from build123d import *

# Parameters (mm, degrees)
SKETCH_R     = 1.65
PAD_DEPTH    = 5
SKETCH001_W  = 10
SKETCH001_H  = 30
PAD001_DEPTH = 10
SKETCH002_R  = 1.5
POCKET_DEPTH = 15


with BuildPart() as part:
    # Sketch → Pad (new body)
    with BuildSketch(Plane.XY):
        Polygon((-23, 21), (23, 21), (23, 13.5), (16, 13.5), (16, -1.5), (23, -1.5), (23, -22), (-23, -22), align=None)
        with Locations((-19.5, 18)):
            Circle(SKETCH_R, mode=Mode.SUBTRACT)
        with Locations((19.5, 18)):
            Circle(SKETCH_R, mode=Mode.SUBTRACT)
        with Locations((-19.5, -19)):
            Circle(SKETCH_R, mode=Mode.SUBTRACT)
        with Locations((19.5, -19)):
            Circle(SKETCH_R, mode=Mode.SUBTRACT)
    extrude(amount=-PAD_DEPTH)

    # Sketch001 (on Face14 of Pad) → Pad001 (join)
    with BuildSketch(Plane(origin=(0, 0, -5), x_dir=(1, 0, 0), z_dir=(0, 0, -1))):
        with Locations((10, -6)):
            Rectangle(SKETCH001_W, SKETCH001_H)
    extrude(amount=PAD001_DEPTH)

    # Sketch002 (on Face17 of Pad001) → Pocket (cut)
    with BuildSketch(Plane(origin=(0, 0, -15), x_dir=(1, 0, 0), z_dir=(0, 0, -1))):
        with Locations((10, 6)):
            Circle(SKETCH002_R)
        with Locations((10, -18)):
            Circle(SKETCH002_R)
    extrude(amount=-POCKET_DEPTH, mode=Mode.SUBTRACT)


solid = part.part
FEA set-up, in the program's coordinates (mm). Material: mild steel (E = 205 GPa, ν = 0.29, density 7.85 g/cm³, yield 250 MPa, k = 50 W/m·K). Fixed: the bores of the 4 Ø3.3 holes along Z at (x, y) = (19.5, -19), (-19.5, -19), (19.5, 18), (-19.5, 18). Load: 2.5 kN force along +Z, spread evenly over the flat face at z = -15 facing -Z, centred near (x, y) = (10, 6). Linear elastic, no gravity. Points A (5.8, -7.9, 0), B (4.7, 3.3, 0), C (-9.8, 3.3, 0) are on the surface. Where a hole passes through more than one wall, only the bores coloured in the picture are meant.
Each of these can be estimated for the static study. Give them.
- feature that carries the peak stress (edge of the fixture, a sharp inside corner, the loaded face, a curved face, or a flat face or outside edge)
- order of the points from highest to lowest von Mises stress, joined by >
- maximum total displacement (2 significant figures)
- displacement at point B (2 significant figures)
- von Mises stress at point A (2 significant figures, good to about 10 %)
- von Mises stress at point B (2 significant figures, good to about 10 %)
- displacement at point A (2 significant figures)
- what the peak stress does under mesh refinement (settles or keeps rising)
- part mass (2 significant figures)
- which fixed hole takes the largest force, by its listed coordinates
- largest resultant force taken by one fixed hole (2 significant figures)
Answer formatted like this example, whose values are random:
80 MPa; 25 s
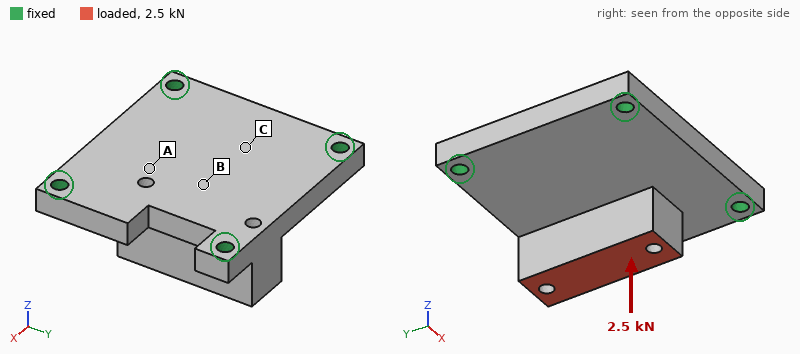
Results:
edge of the fixture; A > B > C; 12 µm; 10 µm; 43 MPa; 33 MPa; 9.8 µm; keeps rising; 94 g; (19.5, 18); 1.4 kN
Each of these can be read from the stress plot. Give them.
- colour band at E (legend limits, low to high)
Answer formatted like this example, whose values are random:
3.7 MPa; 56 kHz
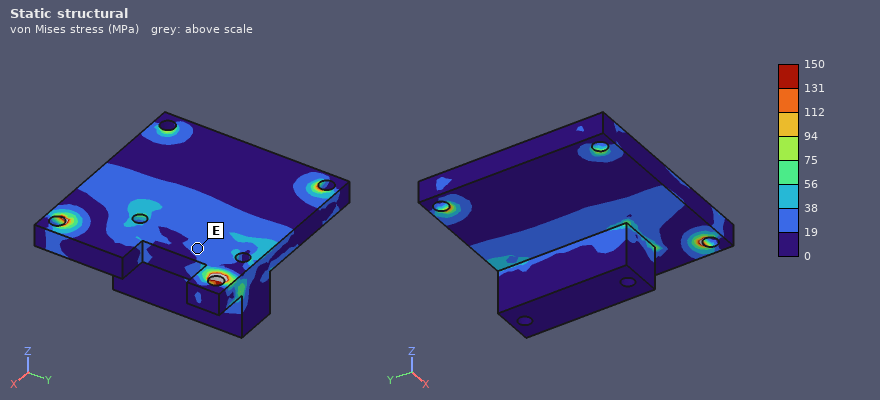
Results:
19 to 38 MPa
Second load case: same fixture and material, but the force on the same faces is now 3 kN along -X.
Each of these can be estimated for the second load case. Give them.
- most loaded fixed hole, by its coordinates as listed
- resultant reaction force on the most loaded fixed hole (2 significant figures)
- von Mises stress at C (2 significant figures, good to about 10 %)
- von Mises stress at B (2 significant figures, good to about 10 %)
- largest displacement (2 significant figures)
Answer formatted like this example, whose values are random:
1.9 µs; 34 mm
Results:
(19.5, 18); 1.4 kN; 23 MPa; 89 MPa; 30 µm
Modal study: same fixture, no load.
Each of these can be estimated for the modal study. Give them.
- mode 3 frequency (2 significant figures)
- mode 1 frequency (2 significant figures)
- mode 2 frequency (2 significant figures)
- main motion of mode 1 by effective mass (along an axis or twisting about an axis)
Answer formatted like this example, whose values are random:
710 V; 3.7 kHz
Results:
19 kHz; 9600 Hz; 15 kHz; along Z
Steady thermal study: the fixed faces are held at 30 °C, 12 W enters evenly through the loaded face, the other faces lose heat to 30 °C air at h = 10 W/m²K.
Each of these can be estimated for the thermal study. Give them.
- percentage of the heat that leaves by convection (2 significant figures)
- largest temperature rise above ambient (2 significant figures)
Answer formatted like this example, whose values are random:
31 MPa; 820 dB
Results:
4.1 %; 24 K
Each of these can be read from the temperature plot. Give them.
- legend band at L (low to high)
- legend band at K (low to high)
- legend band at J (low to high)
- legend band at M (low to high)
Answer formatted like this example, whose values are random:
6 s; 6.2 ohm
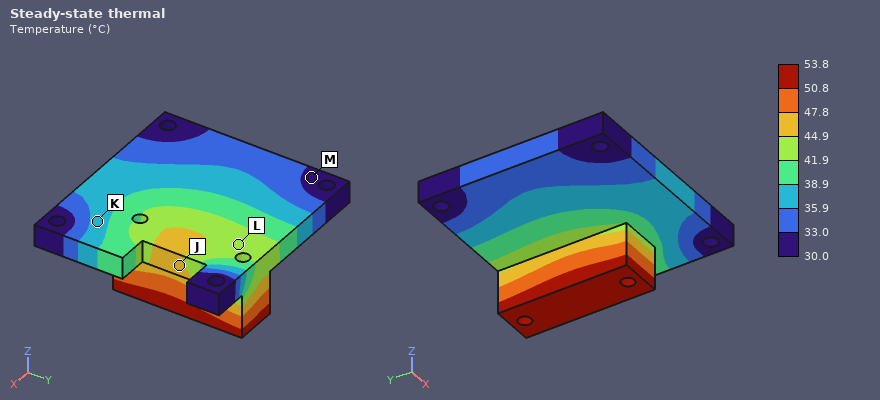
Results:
41.9 to 44.9 °C; 35.9 to 38.9 °C; 44.9 to 47.8 °C; 30.0 to 33.0 °C
